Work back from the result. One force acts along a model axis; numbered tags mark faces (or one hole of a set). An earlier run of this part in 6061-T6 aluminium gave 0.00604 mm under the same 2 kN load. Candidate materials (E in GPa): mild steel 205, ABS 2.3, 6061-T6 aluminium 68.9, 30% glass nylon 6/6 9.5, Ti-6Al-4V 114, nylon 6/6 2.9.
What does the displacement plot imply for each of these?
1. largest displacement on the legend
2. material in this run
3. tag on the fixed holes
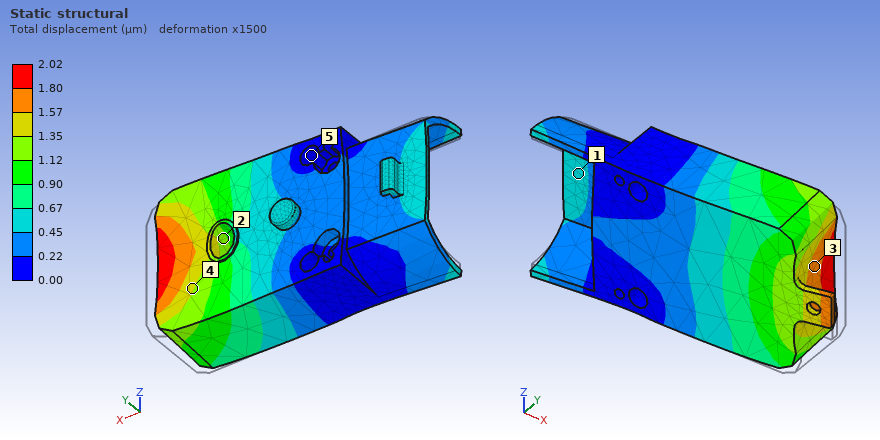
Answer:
2.02 µm
mild steel
5
